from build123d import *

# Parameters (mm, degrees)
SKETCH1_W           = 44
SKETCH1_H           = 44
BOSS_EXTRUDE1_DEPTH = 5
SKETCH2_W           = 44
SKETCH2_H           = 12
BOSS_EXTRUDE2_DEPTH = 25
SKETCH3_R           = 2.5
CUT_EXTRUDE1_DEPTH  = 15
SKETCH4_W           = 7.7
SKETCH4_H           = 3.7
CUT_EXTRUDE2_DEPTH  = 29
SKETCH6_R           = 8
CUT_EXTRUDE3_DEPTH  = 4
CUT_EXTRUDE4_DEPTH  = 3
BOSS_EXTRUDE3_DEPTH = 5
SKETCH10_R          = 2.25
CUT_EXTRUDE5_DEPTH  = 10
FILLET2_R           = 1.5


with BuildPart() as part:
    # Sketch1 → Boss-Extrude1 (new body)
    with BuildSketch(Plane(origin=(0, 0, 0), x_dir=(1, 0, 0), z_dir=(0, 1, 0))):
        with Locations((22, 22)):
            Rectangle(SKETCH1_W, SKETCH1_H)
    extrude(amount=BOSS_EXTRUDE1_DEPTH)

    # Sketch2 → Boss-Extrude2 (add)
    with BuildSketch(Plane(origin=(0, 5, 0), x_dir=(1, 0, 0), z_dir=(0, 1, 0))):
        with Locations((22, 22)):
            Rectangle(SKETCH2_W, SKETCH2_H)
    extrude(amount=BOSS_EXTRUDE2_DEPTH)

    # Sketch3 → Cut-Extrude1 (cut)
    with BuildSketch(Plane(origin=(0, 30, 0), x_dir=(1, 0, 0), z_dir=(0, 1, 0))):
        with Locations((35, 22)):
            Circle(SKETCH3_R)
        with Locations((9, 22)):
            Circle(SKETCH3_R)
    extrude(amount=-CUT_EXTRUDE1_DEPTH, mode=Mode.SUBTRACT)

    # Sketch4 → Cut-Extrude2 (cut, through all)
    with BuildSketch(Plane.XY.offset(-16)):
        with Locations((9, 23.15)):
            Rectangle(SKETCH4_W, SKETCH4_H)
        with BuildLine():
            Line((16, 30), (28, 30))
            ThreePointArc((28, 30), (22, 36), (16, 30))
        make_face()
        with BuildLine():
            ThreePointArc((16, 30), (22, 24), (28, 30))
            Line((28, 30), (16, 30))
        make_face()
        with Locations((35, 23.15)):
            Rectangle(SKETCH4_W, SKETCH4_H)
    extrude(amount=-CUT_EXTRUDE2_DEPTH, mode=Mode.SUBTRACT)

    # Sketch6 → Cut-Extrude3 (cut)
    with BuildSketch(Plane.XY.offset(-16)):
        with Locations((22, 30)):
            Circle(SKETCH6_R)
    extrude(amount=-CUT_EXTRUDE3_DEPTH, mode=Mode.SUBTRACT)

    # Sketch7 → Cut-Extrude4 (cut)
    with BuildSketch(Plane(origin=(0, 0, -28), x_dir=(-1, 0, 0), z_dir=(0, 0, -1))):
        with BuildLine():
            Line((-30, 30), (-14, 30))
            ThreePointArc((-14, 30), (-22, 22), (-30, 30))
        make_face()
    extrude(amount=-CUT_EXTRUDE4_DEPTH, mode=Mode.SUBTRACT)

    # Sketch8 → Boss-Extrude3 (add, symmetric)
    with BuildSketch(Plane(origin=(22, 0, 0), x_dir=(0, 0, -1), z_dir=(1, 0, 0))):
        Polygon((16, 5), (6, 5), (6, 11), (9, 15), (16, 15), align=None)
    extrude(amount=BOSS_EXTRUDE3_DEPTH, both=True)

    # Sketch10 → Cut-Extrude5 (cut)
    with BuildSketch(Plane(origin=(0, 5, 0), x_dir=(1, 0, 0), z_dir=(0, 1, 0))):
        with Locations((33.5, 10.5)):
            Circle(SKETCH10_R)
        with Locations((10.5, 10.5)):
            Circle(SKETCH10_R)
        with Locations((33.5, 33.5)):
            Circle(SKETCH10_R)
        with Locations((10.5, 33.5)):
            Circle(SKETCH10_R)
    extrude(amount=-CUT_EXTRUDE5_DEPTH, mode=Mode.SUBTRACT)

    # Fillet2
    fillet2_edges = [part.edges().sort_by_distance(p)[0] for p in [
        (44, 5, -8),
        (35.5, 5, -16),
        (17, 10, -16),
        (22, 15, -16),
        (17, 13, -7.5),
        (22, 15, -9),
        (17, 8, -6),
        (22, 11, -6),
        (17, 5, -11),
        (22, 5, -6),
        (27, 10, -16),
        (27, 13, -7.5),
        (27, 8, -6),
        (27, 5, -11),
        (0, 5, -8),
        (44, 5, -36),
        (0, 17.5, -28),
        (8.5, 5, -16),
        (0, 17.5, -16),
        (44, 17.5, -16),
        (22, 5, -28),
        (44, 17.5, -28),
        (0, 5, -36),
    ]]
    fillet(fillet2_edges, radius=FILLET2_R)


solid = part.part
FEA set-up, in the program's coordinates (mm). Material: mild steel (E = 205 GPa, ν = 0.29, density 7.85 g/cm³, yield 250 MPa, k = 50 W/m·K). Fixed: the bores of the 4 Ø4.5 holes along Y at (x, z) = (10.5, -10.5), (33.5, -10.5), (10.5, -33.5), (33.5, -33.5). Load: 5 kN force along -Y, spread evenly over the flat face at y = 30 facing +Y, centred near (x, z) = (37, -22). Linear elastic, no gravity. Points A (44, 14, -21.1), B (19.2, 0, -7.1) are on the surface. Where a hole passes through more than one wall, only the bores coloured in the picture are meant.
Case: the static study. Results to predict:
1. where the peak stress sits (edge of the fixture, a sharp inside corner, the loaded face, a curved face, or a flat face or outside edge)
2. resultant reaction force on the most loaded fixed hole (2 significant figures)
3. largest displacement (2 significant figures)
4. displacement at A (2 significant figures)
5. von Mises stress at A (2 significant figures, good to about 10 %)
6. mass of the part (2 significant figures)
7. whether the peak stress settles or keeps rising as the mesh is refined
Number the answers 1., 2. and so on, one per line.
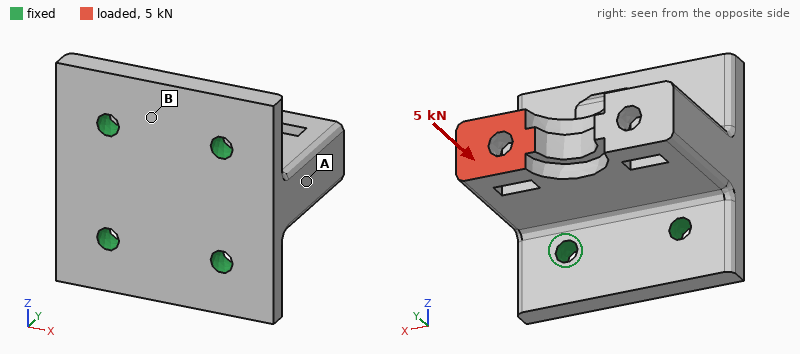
1. edge of the fixture
2. 2.9 kN
3. 15 µm
4. 10.0 µm
5. 44 MPa
6. 170 g
7. keeps rising
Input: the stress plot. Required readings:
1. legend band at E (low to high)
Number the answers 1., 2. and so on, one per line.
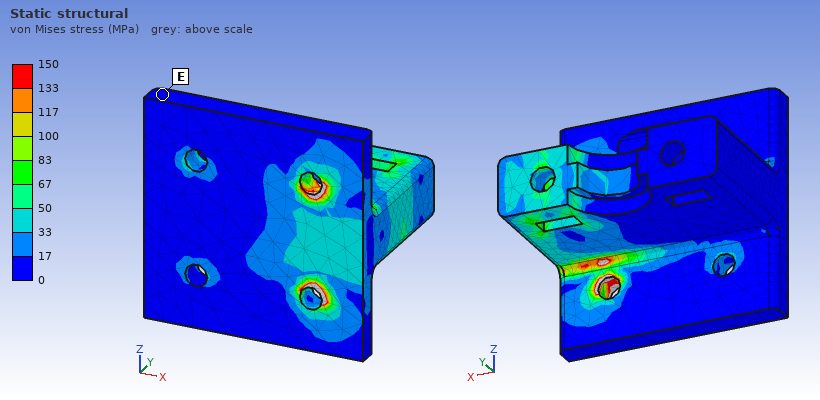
1. 0 to 17 MPa
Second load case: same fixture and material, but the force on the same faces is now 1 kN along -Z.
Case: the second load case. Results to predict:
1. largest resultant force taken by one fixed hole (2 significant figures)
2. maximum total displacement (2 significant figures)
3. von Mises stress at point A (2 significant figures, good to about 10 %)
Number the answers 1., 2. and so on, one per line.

1. 960 N
2. 15 µm
3. 12 MPa
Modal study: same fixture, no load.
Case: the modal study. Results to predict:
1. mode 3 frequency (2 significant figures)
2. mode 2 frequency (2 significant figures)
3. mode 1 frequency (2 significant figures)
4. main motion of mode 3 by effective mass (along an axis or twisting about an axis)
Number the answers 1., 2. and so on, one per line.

1. 17 kHz
2. 13 kHz
3. 12 kHz
4. twisting about Y
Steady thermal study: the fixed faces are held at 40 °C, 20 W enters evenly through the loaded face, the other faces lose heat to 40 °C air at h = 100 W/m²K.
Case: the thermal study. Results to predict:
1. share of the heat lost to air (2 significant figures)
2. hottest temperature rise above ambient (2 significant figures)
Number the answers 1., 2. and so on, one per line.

1. 32 %
2. 55 K
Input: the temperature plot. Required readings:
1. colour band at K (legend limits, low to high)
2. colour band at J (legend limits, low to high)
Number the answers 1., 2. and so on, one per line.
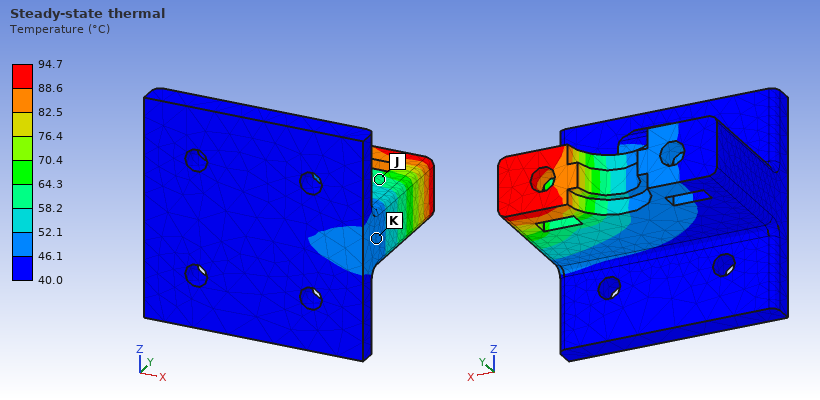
1. 46.1 to 52.1 °C
2. 58.2 to 64.3 °C
